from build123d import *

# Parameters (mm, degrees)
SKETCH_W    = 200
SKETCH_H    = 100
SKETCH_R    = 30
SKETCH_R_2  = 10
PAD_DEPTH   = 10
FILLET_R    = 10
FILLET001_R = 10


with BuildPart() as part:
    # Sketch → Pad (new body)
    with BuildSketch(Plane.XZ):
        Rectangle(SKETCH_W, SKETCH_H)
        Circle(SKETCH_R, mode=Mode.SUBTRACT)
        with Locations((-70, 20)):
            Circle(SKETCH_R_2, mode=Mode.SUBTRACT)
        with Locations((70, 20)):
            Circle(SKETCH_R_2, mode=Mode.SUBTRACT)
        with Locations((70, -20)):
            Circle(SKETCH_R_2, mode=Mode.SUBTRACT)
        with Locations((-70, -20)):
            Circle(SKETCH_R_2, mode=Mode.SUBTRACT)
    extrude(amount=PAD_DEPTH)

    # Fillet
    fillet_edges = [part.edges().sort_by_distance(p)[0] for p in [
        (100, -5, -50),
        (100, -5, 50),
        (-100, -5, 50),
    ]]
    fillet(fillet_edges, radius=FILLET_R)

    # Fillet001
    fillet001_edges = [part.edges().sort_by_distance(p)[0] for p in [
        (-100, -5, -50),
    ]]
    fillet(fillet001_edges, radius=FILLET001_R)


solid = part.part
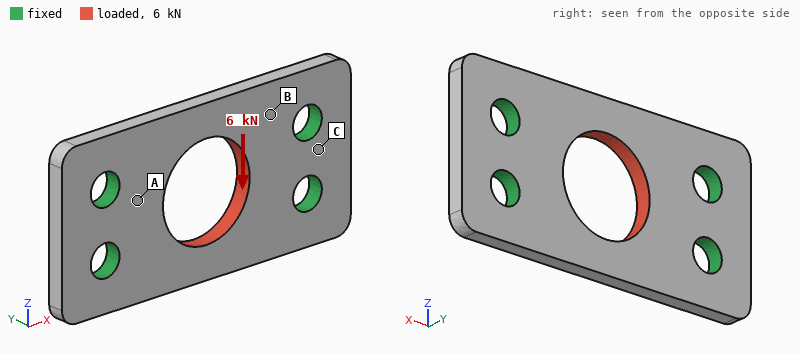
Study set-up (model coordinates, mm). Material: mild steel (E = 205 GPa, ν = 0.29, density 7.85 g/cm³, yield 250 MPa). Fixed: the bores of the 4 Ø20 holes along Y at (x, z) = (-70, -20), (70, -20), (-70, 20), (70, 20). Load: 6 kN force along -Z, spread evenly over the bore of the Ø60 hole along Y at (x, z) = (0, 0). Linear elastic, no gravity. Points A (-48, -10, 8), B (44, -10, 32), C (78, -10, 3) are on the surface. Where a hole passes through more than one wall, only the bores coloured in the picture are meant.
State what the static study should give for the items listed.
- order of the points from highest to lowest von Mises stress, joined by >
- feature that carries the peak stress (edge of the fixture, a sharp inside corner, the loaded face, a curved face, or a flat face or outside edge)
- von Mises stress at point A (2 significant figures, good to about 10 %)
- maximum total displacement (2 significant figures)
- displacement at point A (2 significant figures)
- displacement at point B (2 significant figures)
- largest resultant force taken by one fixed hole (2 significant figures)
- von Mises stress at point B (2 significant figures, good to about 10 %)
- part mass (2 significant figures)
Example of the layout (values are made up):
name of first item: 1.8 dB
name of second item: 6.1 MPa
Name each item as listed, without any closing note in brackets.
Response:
order of the points from highest to lowest von Mises stress, joined by >: A > B > C
feature that carries the peak stress: edge of the fixture
von Mises stress at point A: 8.7 MPa
maximum total displacement: 3.6 µm
displacement at point A: 0.89 µm
displacement at point B: 1.1 µm
largest resultant force taken by one fixed hole: 1.8 kN
von Mises stress at point B: 4.0 MPa
part mass: 1.2 kg
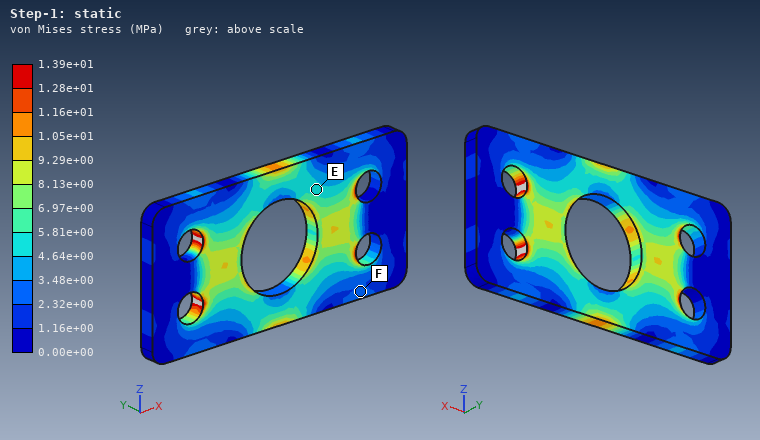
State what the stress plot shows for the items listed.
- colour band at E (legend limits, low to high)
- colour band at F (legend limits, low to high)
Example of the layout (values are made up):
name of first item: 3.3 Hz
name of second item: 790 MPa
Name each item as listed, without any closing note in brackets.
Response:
colour band at E: 4.64e+00 to 5.81e+00 MPa
colour band at F: 2.32e+00 to 3.48e+00 MPa
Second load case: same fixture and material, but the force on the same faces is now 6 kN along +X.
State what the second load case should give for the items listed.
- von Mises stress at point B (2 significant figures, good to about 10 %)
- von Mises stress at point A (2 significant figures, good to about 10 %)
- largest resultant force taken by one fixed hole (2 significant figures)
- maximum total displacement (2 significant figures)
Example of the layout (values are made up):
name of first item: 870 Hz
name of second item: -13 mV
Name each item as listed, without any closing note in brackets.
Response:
von Mises stress at point B: 3.3 MPa
von Mises stress at point A: 3.2 MPa
largest resultant force taken by one fixed hole: 1.5 kN
maximum total displacement: 1.1 µm
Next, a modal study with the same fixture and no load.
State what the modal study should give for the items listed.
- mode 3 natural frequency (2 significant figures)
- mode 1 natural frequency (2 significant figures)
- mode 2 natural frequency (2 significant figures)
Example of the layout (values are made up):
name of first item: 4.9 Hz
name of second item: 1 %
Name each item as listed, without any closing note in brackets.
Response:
mode 3 natural frequency: 7400 Hz
mode 1 natural frequency: 3400 Hz
mode 2 natural frequency: 3500 Hz
